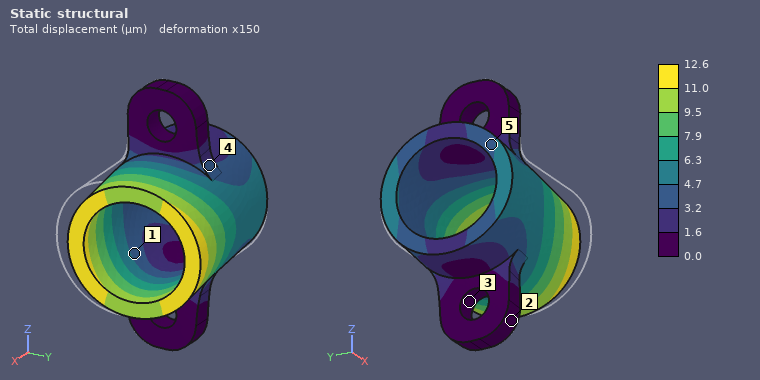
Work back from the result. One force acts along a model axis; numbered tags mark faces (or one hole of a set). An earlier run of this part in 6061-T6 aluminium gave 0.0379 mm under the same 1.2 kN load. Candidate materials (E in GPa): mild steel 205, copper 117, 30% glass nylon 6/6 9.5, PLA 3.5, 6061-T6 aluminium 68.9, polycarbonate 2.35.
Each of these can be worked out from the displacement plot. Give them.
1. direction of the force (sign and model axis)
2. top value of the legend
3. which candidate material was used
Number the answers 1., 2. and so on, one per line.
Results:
1. +Y
2. 12.6 µm
3. mild steel
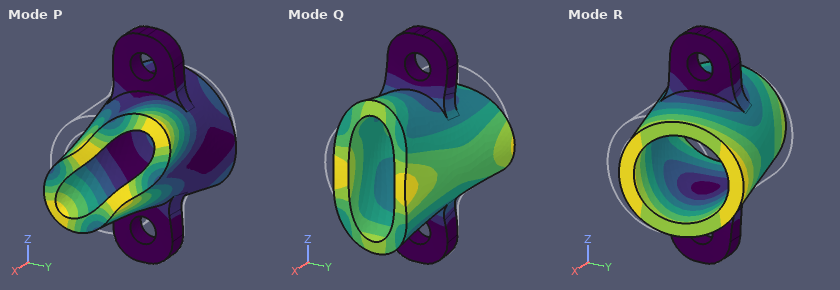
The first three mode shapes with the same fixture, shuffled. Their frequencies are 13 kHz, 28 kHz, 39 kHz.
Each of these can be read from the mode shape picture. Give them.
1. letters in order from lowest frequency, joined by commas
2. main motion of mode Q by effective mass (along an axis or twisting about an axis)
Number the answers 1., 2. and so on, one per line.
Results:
1. R, Q, P
2. along X
